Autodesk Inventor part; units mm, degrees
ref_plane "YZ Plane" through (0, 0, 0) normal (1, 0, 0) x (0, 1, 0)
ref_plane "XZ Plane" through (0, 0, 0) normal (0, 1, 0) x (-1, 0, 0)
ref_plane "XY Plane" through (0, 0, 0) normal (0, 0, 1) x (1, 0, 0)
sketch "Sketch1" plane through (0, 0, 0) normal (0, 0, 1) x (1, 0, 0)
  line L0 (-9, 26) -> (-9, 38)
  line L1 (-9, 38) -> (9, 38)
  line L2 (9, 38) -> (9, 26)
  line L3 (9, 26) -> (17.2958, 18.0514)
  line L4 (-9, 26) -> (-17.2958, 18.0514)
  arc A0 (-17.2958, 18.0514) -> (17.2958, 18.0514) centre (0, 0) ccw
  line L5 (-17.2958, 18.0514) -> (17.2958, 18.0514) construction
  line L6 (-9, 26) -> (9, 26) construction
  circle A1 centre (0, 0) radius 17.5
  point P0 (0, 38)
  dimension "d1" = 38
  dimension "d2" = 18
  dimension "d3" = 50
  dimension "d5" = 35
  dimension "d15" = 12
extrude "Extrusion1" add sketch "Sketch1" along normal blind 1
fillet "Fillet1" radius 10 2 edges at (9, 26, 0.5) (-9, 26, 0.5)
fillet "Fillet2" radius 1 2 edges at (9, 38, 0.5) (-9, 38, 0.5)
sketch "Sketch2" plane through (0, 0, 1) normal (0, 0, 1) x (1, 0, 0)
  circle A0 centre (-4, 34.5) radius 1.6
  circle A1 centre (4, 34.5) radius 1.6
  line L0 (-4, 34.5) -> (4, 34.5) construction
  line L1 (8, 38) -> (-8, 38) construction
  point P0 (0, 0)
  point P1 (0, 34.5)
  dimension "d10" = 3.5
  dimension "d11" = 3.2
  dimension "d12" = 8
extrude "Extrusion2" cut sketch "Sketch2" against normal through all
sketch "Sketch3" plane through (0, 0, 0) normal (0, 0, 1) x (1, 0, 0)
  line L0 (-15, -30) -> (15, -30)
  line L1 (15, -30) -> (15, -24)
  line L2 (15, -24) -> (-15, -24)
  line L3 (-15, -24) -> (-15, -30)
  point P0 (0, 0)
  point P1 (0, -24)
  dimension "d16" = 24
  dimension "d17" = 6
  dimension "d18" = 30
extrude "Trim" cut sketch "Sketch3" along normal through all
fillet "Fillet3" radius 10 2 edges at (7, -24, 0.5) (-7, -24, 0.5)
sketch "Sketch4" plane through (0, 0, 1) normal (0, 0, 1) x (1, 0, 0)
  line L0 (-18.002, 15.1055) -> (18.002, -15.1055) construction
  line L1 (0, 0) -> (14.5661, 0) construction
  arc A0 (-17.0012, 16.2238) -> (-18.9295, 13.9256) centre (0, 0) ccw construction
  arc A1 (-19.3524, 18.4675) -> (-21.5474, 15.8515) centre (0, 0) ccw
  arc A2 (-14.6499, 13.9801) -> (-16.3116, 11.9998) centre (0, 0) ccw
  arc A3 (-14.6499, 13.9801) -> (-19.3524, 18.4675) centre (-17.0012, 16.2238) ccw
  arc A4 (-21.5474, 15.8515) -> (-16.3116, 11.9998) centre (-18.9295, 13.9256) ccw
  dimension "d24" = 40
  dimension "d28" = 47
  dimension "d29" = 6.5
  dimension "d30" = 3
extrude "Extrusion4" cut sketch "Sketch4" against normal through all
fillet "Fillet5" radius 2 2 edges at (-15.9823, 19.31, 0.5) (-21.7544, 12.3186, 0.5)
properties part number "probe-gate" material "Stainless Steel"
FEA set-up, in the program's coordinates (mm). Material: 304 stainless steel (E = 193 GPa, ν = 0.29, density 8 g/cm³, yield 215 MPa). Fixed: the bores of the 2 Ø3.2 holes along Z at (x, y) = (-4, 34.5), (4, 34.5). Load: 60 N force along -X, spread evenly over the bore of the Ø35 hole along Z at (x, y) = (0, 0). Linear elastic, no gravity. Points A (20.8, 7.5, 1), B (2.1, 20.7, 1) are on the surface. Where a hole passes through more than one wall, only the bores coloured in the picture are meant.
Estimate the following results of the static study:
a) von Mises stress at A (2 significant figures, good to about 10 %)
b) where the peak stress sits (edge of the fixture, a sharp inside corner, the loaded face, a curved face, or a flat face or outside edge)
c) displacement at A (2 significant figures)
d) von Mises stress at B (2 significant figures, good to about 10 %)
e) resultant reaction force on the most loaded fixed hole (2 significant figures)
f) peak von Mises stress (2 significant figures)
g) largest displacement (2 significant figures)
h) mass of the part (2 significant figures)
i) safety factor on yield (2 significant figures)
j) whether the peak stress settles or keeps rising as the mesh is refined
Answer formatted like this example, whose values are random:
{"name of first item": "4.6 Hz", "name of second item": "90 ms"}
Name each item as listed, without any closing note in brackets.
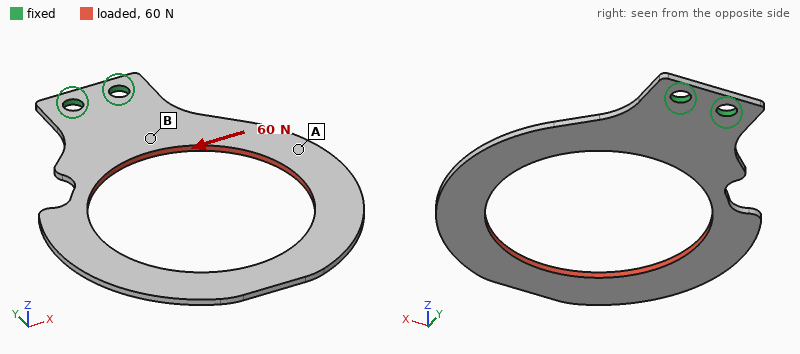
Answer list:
{"von Mises stress at A": "9.1 MPa", "where the peak stress sits": "a curved face", "displacement at A": "23 µm", "von Mises stress at B": "23 MPa", "resultant reaction force on the most loaded fixed hole": "200 N", "peak von Mises stress": "90 MPa", "largest displacement": "53 µm", "mass of the part": "9.6 g", "safety factor on yield": "2.4", "whether the peak stress settles or keeps rising as the mesh is refined": "settles"}
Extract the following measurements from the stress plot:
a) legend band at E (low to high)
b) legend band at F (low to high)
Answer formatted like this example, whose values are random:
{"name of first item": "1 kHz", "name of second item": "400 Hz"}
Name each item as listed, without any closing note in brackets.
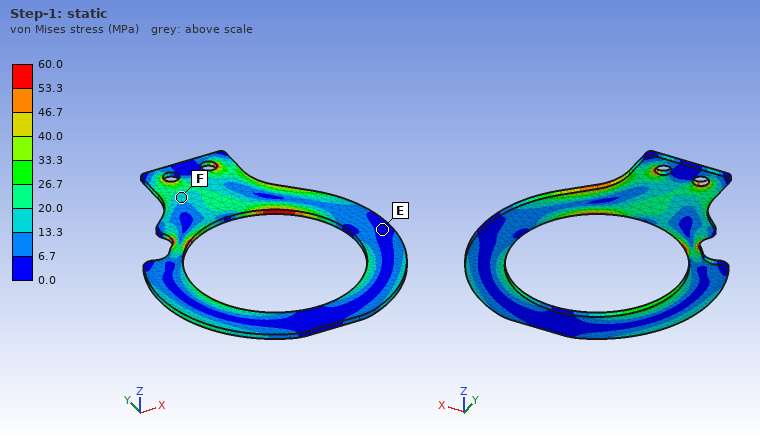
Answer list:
{"legend band at E": "0.0 to 6.7 MPa", "legend band at F": "13.3 to 20.0 MPa"}
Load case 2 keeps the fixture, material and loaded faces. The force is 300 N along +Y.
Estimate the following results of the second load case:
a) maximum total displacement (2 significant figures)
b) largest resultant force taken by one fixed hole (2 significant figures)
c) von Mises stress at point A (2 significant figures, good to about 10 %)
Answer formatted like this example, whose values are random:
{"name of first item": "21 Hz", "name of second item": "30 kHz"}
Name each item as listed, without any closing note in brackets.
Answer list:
{"maximum total displacement": "28 µm", "largest resultant force taken by one fixed hole": "150 N", "von Mises stress at point A": "8.1 MPa"}
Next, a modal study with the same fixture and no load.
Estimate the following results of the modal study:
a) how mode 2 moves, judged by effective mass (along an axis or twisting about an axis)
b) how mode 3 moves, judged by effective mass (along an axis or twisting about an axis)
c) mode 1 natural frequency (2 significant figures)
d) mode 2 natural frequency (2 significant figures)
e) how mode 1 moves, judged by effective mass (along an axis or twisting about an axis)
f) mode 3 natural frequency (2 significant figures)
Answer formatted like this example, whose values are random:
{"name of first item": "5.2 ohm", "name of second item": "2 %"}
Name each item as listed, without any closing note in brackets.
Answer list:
{"how mode 2 moves, judged by effective mass": "twisting about Y", "how mode 3 moves, judged by effective mass": "along Z", "mode 1 natural frequency": "200 Hz", "mode 2 natural frequency": "460 Hz", "how mode 1 moves, judged by effective mass": "along Z", "mode 3 natural frequency": "1100 Hz"}
